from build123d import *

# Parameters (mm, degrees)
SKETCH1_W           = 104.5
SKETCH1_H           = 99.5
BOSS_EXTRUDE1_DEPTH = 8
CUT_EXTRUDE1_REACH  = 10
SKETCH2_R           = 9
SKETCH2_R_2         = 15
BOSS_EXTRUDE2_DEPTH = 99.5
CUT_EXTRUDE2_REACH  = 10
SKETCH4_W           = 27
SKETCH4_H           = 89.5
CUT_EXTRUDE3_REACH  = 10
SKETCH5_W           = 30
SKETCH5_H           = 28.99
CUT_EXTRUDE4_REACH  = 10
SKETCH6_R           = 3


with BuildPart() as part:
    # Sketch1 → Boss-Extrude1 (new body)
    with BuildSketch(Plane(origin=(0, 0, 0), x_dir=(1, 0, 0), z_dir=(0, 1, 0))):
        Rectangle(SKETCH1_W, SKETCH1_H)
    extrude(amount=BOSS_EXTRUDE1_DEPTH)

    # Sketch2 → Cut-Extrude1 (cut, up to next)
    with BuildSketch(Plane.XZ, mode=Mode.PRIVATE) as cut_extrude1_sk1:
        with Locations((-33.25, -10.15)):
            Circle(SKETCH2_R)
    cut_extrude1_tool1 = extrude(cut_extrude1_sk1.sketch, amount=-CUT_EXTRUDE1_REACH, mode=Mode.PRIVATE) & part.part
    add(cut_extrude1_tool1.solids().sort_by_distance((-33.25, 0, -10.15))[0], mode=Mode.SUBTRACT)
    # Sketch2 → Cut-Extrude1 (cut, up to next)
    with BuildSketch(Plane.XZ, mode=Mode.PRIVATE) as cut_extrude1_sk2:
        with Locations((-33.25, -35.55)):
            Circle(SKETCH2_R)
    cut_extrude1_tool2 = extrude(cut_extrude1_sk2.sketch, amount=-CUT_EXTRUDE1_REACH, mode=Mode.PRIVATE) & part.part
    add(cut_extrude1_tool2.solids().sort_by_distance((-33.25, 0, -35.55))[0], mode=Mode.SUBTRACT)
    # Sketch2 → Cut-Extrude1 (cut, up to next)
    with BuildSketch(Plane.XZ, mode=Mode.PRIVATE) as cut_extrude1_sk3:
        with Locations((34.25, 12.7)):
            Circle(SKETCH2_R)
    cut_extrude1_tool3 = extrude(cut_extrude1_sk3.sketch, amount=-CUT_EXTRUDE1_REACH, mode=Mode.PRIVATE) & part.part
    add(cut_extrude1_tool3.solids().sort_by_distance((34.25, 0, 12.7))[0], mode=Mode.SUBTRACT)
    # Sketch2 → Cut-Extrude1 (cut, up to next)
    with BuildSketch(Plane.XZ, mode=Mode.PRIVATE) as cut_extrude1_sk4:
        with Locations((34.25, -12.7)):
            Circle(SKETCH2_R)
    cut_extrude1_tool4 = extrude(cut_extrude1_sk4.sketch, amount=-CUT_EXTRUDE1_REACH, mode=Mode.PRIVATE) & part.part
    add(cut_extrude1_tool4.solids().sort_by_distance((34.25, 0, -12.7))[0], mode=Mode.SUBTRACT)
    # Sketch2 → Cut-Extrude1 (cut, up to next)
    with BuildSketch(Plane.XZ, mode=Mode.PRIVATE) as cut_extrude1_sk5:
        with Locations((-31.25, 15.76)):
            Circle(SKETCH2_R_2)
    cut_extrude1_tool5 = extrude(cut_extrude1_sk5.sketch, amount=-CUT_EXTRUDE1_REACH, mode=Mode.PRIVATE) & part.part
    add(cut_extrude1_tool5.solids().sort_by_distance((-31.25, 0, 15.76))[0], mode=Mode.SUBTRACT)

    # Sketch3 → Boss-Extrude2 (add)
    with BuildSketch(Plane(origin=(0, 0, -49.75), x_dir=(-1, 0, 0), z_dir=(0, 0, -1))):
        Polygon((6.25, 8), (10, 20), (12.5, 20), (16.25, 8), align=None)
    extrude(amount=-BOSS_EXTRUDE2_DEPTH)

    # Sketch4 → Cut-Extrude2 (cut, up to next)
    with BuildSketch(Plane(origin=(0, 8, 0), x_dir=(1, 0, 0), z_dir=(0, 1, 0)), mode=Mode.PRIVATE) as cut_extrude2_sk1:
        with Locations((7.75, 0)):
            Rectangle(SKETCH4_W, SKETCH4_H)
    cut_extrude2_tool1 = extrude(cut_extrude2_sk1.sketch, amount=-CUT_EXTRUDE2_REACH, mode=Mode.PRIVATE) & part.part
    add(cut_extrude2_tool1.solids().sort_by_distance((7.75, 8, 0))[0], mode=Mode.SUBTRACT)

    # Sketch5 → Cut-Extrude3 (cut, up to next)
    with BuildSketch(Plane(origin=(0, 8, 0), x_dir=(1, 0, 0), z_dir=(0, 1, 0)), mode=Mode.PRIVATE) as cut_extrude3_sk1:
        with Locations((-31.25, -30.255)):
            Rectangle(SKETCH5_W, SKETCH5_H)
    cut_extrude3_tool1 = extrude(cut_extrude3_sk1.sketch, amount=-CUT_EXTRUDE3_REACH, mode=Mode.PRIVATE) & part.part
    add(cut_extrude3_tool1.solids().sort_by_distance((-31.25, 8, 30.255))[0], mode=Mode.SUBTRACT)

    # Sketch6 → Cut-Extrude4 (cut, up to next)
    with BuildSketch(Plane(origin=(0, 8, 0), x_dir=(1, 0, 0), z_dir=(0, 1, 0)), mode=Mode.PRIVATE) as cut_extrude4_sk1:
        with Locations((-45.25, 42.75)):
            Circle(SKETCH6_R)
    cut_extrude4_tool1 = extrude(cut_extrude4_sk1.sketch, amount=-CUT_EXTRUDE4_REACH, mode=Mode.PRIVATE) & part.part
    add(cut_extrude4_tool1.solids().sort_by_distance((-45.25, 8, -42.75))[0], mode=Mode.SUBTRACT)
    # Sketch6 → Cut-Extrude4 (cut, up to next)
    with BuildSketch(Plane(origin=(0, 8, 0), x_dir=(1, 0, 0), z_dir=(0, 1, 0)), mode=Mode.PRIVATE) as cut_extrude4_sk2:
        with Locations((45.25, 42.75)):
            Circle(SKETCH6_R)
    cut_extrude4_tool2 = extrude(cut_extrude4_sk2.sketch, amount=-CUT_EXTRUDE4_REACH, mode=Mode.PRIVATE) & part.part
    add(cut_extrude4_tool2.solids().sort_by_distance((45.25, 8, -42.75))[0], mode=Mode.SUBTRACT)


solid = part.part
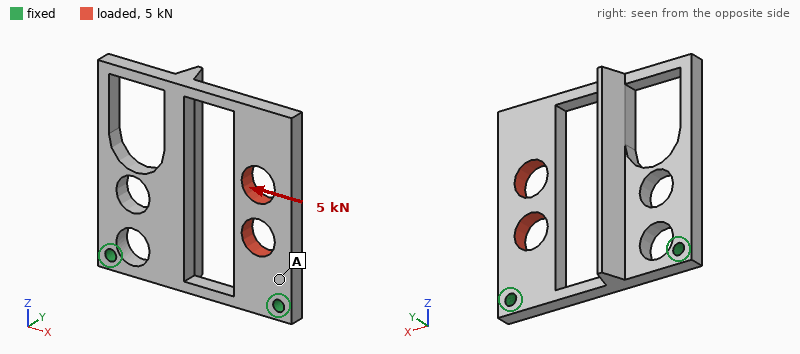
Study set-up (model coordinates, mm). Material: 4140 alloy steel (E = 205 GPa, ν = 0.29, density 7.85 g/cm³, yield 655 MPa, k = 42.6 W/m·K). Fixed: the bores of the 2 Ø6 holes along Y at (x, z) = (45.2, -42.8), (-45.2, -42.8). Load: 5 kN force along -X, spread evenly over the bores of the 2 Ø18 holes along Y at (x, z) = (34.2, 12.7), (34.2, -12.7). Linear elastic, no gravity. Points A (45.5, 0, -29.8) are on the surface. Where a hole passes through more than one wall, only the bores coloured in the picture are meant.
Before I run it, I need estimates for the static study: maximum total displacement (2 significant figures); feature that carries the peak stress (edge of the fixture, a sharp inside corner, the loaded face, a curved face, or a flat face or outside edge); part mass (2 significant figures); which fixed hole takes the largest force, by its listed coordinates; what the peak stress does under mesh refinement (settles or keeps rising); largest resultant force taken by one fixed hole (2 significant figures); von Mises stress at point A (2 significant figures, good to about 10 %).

0.15 mm
edge of the fixture
420 g
(45.2, -42.8)
keeps rising
4.5 kN
37 MPa
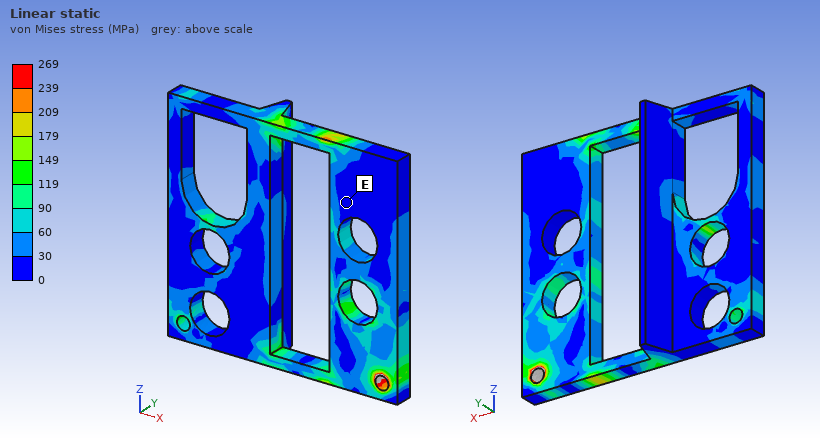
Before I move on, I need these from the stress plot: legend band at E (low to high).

0 to 30 MPa
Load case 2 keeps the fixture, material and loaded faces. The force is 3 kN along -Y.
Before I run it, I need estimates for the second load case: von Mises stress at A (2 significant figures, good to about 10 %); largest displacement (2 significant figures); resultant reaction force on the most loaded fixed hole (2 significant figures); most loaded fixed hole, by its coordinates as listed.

230 MPa
0.70 mm
2.8 kN
(45.2, -42.8)
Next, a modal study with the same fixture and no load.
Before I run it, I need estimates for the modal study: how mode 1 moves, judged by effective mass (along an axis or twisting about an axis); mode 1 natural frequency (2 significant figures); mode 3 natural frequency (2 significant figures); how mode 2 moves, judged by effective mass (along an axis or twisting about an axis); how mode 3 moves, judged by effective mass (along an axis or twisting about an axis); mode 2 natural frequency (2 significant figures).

along Y
600 Hz
1700 Hz
twisting about Z
along X
1400 Hz
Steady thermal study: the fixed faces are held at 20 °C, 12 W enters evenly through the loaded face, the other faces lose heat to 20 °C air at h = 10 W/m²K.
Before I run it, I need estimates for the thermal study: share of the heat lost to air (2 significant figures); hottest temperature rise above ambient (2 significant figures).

25 %
48 K
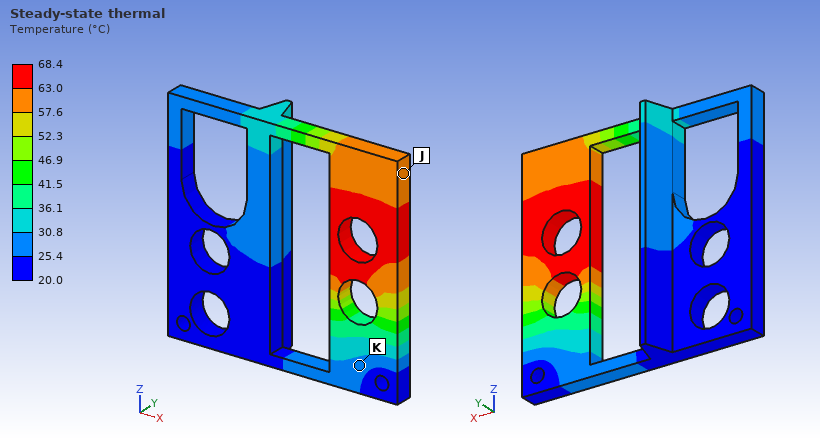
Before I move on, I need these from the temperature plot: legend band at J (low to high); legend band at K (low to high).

57.6 to 63.0 °C
25.4 to 30.8 °C
